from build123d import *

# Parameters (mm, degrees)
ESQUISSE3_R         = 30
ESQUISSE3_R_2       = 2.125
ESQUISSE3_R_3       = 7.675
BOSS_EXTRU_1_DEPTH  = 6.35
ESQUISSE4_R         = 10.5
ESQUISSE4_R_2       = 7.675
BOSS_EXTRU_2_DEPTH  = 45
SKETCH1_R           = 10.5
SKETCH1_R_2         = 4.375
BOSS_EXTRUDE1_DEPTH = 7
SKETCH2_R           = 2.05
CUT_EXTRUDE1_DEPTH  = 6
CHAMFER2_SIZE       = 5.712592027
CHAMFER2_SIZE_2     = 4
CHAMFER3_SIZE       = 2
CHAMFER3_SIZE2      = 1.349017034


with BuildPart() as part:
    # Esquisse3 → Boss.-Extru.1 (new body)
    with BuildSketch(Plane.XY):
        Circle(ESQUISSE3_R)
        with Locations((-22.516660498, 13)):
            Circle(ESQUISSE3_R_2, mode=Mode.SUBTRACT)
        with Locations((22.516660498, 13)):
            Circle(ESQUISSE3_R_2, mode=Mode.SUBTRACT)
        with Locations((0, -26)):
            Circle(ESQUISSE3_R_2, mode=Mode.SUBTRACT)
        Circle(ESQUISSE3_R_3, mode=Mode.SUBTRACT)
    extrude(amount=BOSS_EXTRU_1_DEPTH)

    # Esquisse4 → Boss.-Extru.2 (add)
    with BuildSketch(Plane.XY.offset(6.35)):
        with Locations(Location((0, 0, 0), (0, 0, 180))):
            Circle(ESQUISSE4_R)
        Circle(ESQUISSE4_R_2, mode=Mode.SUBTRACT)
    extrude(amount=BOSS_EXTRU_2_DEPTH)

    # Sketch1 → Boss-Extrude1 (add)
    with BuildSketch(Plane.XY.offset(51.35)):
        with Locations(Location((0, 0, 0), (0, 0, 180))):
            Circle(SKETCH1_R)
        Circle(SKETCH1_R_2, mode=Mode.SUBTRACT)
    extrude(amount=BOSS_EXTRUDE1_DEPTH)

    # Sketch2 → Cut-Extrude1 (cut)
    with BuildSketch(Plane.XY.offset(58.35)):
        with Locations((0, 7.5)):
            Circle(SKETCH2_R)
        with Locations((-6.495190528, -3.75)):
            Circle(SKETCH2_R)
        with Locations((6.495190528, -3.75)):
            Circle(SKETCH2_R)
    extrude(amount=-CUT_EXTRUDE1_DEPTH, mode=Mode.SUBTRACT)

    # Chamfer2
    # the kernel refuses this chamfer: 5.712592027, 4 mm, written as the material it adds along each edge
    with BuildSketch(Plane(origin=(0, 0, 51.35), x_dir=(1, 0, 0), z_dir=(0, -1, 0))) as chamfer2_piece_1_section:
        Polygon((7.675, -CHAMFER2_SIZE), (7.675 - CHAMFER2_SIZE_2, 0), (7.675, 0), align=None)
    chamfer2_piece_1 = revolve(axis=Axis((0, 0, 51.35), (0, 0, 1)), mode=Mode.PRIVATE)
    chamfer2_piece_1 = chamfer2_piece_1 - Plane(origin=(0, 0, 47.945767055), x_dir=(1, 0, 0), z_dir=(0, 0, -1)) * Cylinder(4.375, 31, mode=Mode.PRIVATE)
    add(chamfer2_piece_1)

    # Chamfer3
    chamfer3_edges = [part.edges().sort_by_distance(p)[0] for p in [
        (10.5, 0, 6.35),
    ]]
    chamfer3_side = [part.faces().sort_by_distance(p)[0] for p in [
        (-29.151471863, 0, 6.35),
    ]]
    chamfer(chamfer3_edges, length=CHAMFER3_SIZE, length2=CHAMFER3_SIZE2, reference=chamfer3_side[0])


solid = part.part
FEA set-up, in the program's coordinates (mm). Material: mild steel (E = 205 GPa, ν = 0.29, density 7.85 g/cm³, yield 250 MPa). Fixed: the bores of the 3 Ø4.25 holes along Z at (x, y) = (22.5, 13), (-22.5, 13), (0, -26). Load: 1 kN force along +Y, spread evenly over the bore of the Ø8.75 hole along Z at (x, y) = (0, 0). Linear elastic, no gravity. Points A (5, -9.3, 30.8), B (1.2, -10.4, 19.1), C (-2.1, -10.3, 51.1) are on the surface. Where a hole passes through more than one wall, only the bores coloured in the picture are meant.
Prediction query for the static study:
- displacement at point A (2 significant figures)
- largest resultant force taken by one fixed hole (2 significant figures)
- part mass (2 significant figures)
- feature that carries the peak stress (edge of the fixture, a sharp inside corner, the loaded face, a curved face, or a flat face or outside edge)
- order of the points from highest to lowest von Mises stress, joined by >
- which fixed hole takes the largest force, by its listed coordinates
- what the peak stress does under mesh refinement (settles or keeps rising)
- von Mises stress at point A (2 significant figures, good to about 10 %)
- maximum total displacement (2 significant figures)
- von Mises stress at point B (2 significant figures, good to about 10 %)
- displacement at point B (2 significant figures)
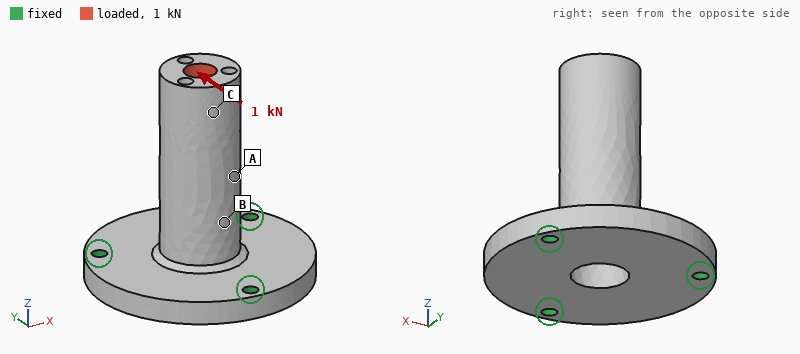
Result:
34 µm
1.5 kN
200 g
edge of the fixture
B > A > C
(0, -26)
keeps rising
33 MPa
78 µm
51 MPa
19 µm
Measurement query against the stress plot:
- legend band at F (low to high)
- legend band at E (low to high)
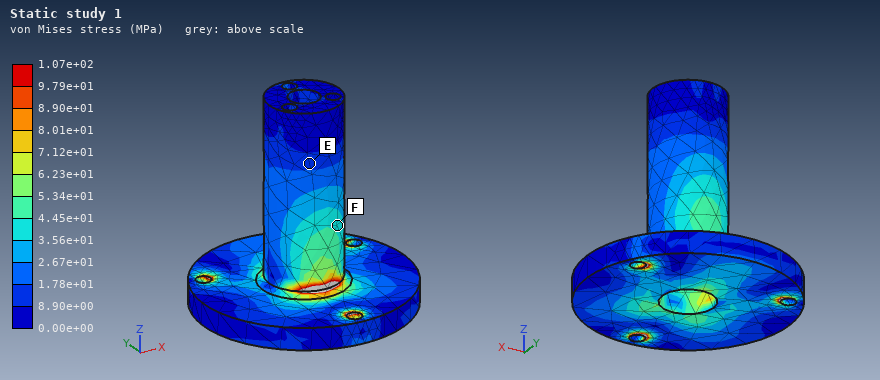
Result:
3.56e+01 to 4.45e+01 MPa
8.90e+00 to 1.78e+01 MPa
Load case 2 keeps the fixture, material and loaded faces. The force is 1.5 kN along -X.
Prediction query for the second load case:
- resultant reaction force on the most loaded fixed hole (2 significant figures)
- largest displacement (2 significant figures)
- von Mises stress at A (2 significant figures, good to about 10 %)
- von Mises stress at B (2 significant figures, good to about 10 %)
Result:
1.9 kN
0.12 mm
37 MPa
28 MPa
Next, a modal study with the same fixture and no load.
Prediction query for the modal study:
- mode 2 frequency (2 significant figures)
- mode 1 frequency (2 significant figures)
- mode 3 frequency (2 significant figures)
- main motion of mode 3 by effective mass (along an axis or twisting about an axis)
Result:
3300 Hz
3300 Hz
8600 Hz
along Z
